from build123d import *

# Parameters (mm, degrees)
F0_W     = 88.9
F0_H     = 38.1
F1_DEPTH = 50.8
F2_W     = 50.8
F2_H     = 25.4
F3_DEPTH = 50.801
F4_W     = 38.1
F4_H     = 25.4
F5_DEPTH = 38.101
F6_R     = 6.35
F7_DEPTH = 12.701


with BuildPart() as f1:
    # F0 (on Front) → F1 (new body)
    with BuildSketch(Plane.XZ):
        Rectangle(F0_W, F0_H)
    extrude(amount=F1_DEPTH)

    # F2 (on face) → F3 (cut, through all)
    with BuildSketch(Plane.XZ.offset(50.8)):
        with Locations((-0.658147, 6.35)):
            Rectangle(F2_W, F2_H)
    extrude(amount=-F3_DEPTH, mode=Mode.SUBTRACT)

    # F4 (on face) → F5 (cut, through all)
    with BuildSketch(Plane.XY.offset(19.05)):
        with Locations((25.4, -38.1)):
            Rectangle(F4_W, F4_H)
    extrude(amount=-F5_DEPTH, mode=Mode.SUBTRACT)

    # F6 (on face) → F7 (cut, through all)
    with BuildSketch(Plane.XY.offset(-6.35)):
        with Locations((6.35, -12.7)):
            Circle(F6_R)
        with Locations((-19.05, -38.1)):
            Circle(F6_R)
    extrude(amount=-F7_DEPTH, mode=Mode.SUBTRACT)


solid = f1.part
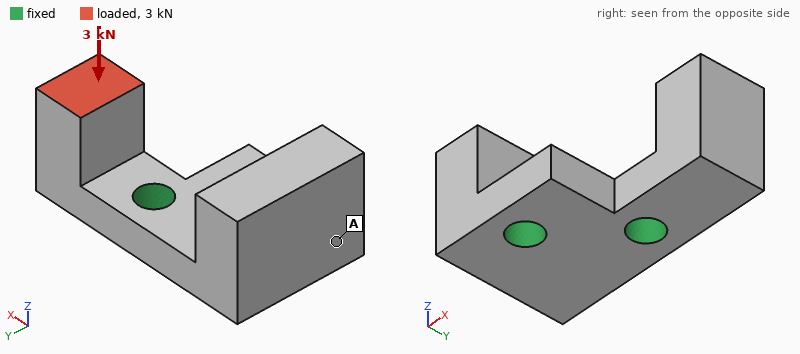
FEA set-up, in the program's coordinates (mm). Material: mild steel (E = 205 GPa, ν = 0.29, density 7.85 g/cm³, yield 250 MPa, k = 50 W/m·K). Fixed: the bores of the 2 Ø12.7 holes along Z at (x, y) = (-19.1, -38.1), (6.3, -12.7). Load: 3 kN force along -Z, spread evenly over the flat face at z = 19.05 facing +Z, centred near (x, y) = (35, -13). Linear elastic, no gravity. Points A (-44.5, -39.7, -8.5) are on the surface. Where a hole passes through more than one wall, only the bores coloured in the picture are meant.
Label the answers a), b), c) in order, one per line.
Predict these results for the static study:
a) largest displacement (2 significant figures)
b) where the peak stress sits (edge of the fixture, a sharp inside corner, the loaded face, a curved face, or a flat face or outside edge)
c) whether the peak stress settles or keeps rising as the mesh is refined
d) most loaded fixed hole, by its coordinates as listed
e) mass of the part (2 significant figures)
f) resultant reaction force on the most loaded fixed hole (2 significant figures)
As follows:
a) 43 µm
b) edge of the fixture
c) keeps rising
d) (6.3, -12.7)
e) 610 g
f) 3.1 kN
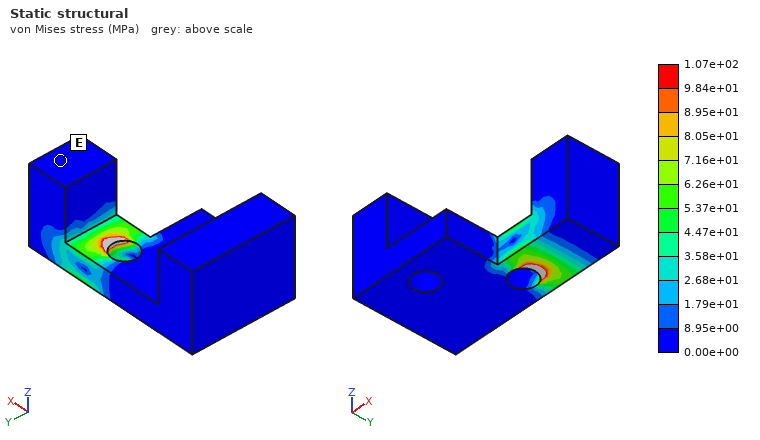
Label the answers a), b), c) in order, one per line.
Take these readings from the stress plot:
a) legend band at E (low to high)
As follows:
a) 0.00e+00 to 8.95e+00 MPa
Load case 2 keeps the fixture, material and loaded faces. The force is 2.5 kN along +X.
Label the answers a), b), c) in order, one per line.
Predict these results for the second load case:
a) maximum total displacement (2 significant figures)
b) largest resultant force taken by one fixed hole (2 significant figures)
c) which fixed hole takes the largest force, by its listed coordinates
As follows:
a) 79 µm
b) 2.4 kN
c) (6.3, -12.7)
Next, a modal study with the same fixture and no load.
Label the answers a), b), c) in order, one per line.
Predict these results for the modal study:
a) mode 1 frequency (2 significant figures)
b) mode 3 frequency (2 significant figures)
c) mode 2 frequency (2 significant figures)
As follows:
a) 3600 Hz
b) 4800 Hz
c) 4700 Hz
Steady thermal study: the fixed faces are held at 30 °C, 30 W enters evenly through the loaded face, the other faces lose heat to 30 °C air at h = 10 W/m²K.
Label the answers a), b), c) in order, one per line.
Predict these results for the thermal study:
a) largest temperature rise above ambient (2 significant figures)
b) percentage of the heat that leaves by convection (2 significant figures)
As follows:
a) 68 K
b) 6.1 %
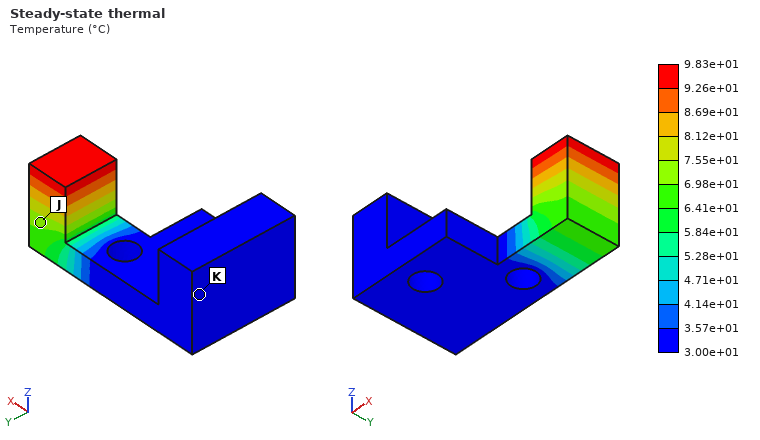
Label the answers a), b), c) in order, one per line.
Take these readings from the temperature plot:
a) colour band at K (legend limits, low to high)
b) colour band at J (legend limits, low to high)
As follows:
a) 3.00e+01 to 3.57e+01 °C
b) 6.98e+01 to 7.55e+01 °C
